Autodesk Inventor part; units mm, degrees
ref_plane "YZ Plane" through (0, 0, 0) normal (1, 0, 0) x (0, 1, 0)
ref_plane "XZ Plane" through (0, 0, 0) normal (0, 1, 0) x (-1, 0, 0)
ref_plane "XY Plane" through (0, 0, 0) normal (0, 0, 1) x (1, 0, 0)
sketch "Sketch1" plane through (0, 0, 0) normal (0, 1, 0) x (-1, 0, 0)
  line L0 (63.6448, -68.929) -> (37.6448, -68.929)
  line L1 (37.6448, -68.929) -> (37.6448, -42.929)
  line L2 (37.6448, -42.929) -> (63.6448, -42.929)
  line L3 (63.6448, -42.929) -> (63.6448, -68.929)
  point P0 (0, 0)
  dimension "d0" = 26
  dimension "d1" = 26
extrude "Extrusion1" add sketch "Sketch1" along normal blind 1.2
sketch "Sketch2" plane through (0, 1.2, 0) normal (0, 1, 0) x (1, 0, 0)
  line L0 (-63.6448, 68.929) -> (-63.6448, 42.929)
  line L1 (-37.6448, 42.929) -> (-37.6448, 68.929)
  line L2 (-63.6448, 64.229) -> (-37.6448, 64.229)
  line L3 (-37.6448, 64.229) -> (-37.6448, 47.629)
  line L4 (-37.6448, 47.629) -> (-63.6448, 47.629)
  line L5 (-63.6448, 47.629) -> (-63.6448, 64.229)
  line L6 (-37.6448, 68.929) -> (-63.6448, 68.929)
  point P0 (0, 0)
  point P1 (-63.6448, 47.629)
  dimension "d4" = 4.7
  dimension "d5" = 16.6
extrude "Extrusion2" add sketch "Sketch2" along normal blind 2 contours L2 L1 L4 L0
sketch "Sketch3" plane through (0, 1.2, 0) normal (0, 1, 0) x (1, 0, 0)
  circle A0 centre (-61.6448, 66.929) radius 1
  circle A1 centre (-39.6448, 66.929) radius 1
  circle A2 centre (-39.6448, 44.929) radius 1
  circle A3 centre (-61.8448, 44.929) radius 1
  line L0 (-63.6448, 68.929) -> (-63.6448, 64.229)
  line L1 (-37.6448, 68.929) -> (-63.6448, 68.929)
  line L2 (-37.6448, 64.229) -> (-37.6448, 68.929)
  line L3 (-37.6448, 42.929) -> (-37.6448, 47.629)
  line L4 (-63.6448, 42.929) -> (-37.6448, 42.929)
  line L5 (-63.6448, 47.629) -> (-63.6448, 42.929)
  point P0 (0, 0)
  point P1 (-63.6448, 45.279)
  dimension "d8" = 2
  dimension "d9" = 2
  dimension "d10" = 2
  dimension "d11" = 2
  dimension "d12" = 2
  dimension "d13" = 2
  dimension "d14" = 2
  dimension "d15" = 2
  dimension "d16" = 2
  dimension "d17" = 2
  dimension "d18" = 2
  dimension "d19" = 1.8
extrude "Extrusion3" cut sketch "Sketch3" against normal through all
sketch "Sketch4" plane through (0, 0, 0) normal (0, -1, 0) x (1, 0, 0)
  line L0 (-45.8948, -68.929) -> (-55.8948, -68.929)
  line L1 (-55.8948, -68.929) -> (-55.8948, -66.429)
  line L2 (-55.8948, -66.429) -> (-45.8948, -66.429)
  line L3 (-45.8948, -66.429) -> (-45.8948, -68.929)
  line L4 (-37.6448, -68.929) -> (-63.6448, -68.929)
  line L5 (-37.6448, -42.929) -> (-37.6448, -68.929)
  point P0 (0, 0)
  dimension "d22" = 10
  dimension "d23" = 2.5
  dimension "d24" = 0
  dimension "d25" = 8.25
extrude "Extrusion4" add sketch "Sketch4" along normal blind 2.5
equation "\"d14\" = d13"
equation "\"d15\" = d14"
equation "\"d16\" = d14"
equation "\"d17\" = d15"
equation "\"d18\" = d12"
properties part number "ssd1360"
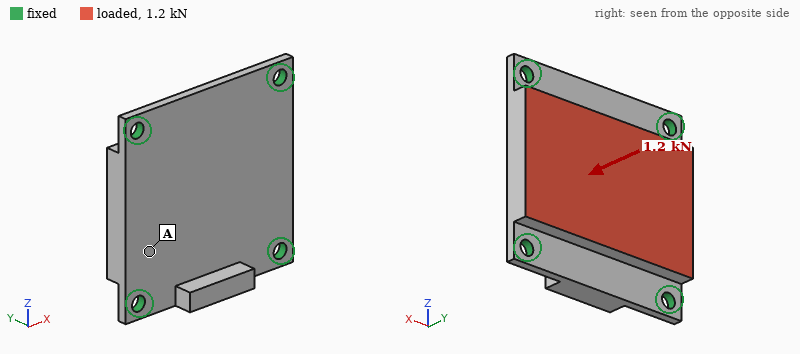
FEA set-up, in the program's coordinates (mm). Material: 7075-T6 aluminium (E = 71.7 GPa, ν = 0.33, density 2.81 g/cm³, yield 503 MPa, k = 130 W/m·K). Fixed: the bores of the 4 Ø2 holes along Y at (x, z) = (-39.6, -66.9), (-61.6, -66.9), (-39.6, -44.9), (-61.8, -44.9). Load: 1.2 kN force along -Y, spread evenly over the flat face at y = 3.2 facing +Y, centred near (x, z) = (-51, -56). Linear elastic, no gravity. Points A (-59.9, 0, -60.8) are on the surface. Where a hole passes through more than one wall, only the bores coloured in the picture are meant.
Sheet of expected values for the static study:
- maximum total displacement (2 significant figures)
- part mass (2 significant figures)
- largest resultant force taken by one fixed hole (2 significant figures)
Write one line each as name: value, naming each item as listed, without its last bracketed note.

maximum total displacement: 45 µm
part mass: 4.8 g
largest resultant force taken by one fixed hole: 450 N
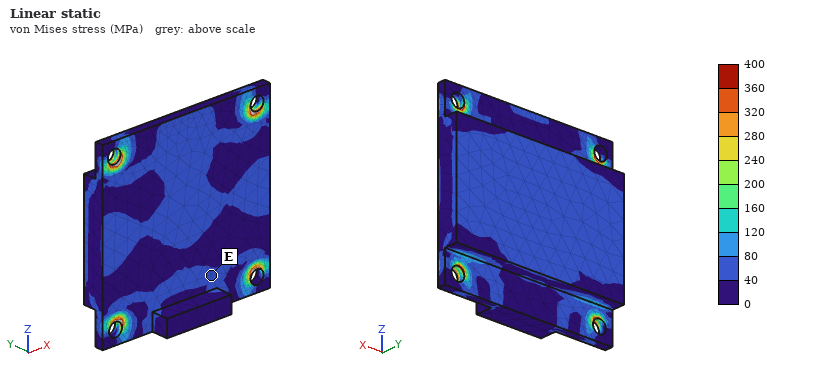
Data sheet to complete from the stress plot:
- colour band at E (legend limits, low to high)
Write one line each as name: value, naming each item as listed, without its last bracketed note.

colour band at E: 40 to 80 MPa
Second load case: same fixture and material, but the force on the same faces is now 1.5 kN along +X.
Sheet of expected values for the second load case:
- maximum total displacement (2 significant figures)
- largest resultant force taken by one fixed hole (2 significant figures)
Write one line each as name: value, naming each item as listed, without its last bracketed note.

maximum total displacement: 15 µm
largest resultant force taken by one fixed hole: 440 N
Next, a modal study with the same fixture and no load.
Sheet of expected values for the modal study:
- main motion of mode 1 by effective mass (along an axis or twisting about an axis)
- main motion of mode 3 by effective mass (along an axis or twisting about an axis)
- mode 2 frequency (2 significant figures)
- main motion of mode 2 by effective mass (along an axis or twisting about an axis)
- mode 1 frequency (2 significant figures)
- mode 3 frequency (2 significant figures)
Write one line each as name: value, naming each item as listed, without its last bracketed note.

main motion of mode 1 by effective mass: along Y
main motion of mode 3 by effective mass: twisting about Z
mode 2 frequency: 20 kHz
main motion of mode 2 by effective mass: twisting about X
mode 1 frequency: 14 kHz
mode 3 frequency: 23 kHz
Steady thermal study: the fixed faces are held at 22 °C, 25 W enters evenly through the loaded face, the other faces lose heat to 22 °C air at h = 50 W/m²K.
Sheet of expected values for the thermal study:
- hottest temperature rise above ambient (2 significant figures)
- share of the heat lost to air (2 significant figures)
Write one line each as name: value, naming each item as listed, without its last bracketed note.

hottest temperature rise above ambient: 26 K
share of the heat lost to air: 4.4 %
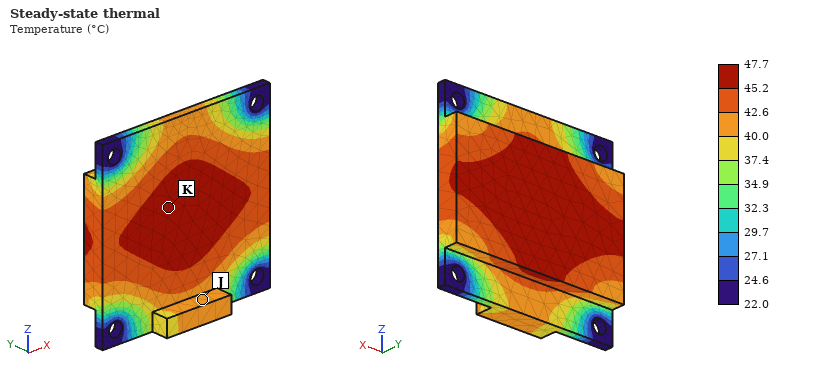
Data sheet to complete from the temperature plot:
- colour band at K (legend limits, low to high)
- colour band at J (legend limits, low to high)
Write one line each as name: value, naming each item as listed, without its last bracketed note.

colour band at K: 45.2 to 47.7 °C
colour band at J: 40.0 to 42.6 °C
